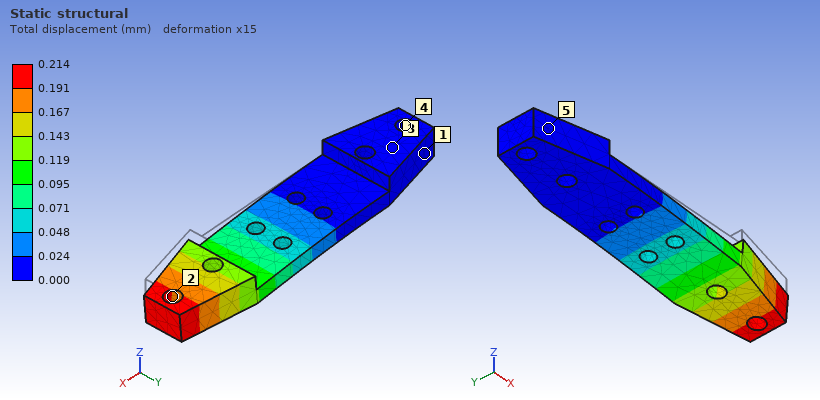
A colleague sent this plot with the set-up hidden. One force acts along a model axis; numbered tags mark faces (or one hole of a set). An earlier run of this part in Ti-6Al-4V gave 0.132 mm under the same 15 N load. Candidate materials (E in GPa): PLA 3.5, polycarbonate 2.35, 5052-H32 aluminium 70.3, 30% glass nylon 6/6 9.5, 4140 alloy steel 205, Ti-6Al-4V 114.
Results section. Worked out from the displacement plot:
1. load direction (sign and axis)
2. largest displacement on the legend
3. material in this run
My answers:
-Z
0.214 mm
5052-H32 aluminium
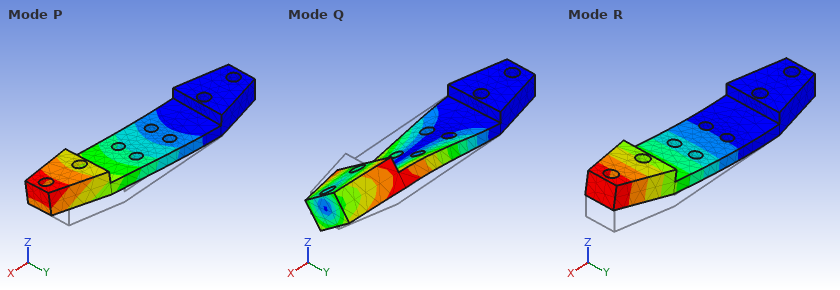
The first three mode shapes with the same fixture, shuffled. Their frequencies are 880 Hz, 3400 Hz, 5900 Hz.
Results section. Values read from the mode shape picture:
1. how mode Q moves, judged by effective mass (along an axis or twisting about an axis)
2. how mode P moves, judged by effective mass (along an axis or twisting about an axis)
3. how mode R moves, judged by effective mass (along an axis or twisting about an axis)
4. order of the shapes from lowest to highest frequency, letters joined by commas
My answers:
twisting about X
along Y
along Z
R, P, Q
